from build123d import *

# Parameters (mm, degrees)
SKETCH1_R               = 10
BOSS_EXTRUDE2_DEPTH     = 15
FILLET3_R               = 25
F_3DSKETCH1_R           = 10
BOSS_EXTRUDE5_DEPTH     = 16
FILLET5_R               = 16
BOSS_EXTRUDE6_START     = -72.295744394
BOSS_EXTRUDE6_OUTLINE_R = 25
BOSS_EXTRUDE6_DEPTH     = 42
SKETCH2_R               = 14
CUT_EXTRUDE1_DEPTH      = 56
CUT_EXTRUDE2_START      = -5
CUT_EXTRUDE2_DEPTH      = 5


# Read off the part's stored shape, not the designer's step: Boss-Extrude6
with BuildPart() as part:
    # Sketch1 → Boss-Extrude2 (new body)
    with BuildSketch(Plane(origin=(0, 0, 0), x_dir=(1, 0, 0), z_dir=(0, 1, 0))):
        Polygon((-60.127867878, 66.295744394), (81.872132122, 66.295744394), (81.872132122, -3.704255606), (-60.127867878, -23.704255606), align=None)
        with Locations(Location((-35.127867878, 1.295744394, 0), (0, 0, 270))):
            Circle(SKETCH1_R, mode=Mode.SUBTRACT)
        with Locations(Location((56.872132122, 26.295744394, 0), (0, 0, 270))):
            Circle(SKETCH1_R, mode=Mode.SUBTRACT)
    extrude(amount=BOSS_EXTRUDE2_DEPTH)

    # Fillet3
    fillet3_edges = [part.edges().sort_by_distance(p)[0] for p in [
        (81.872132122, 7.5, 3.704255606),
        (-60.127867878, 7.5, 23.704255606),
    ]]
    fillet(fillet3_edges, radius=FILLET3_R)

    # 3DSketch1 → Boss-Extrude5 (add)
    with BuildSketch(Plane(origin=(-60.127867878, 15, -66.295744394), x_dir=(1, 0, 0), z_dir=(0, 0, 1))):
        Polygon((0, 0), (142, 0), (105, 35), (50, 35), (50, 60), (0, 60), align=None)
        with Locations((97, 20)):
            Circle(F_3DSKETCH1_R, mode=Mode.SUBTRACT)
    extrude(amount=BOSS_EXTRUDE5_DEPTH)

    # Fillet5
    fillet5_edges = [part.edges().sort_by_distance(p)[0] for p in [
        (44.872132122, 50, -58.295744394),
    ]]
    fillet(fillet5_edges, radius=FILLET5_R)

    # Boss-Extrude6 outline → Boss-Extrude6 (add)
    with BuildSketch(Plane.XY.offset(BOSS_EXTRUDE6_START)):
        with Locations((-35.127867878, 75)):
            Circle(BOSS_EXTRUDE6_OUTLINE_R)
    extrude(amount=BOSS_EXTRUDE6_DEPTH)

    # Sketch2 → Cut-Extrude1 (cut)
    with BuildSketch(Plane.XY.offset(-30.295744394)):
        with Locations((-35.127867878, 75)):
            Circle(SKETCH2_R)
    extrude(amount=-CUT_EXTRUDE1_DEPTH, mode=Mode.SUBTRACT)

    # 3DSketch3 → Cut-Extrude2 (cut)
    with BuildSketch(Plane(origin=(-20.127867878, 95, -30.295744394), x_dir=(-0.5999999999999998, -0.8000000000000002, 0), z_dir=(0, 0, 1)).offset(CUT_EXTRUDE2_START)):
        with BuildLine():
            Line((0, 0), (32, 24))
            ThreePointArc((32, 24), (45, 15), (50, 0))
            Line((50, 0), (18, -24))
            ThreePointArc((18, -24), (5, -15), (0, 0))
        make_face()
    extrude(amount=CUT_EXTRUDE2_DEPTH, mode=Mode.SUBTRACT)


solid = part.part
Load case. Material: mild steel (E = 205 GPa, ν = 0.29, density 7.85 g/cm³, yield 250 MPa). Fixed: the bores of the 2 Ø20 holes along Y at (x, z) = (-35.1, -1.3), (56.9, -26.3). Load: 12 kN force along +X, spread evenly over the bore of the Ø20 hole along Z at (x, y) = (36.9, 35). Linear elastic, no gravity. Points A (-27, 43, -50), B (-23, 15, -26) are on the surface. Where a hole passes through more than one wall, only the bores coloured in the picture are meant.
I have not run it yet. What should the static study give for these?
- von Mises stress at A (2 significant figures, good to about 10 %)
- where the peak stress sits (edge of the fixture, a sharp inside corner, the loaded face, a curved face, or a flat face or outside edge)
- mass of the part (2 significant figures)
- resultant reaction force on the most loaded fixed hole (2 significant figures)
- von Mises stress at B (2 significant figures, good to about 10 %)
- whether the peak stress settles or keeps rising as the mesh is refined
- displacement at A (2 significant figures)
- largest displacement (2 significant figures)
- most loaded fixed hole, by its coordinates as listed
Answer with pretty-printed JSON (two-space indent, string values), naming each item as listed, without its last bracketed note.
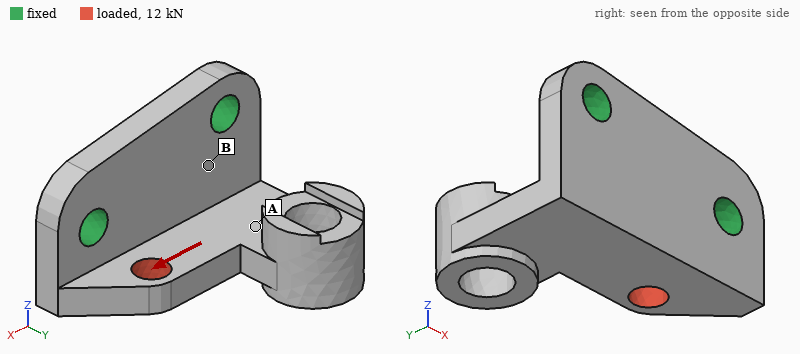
{
  "von Mises stress at A": "7.6 MPa",
  "where the peak stress sits": "edge of the fixture",
  "mass of the part": "2.2 kg",
  "resultant reaction force on the most loaded fixed hole": "9.8 kN",
  "von Mises stress at B": "24 MPa",
  "whether the peak stress settles or keeps rising as the mesh is refined": "keeps rising",
  "displacement at A": "27 µm",
  "largest displacement": "58 µm",
  "most loaded fixed hole, by its coordinates as listed": "(56.9, -26.3)"
}
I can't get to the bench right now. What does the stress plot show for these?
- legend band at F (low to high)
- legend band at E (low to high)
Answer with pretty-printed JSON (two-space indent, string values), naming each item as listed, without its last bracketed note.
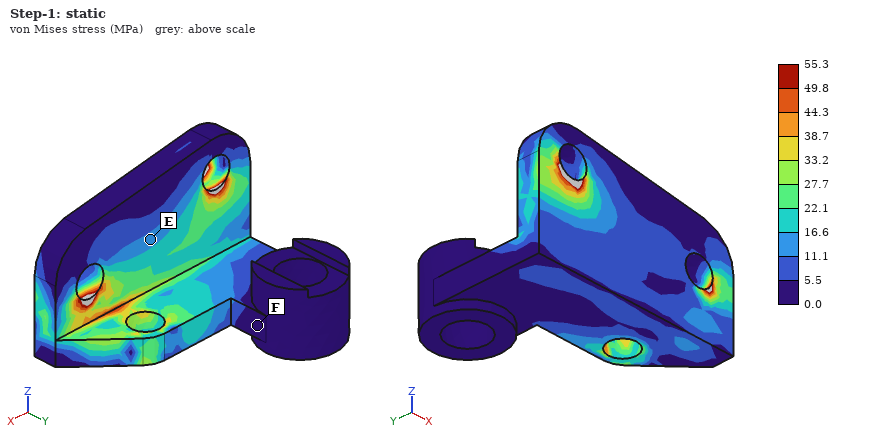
{
  "legend band at F": "0.0 to 5.5 MPa",
  "legend band at E": "11.1 to 16.6 MPa"
}
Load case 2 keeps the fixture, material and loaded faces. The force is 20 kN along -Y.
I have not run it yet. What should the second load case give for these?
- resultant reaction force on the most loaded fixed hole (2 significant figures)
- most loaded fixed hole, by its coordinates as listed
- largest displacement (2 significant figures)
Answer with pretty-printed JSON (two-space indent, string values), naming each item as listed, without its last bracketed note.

{
  "resultant reaction force on the most loaded fixed hole": "17 kN",
  "most loaded fixed hole, by its coordinates as listed": "(56.9, -26.3)",
  "largest displacement": "0.15 mm"
}
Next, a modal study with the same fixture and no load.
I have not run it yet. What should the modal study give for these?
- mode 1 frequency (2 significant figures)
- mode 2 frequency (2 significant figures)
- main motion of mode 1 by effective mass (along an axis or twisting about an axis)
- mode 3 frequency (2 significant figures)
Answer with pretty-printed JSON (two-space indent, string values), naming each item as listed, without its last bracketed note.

{
  "mode 1 frequency": "970 Hz",
  "mode 2 frequency": "2000 Hz",
  "main motion of mode 1 by effective mass": "along Z",
  "mode 3 frequency": "3200 Hz"
}
